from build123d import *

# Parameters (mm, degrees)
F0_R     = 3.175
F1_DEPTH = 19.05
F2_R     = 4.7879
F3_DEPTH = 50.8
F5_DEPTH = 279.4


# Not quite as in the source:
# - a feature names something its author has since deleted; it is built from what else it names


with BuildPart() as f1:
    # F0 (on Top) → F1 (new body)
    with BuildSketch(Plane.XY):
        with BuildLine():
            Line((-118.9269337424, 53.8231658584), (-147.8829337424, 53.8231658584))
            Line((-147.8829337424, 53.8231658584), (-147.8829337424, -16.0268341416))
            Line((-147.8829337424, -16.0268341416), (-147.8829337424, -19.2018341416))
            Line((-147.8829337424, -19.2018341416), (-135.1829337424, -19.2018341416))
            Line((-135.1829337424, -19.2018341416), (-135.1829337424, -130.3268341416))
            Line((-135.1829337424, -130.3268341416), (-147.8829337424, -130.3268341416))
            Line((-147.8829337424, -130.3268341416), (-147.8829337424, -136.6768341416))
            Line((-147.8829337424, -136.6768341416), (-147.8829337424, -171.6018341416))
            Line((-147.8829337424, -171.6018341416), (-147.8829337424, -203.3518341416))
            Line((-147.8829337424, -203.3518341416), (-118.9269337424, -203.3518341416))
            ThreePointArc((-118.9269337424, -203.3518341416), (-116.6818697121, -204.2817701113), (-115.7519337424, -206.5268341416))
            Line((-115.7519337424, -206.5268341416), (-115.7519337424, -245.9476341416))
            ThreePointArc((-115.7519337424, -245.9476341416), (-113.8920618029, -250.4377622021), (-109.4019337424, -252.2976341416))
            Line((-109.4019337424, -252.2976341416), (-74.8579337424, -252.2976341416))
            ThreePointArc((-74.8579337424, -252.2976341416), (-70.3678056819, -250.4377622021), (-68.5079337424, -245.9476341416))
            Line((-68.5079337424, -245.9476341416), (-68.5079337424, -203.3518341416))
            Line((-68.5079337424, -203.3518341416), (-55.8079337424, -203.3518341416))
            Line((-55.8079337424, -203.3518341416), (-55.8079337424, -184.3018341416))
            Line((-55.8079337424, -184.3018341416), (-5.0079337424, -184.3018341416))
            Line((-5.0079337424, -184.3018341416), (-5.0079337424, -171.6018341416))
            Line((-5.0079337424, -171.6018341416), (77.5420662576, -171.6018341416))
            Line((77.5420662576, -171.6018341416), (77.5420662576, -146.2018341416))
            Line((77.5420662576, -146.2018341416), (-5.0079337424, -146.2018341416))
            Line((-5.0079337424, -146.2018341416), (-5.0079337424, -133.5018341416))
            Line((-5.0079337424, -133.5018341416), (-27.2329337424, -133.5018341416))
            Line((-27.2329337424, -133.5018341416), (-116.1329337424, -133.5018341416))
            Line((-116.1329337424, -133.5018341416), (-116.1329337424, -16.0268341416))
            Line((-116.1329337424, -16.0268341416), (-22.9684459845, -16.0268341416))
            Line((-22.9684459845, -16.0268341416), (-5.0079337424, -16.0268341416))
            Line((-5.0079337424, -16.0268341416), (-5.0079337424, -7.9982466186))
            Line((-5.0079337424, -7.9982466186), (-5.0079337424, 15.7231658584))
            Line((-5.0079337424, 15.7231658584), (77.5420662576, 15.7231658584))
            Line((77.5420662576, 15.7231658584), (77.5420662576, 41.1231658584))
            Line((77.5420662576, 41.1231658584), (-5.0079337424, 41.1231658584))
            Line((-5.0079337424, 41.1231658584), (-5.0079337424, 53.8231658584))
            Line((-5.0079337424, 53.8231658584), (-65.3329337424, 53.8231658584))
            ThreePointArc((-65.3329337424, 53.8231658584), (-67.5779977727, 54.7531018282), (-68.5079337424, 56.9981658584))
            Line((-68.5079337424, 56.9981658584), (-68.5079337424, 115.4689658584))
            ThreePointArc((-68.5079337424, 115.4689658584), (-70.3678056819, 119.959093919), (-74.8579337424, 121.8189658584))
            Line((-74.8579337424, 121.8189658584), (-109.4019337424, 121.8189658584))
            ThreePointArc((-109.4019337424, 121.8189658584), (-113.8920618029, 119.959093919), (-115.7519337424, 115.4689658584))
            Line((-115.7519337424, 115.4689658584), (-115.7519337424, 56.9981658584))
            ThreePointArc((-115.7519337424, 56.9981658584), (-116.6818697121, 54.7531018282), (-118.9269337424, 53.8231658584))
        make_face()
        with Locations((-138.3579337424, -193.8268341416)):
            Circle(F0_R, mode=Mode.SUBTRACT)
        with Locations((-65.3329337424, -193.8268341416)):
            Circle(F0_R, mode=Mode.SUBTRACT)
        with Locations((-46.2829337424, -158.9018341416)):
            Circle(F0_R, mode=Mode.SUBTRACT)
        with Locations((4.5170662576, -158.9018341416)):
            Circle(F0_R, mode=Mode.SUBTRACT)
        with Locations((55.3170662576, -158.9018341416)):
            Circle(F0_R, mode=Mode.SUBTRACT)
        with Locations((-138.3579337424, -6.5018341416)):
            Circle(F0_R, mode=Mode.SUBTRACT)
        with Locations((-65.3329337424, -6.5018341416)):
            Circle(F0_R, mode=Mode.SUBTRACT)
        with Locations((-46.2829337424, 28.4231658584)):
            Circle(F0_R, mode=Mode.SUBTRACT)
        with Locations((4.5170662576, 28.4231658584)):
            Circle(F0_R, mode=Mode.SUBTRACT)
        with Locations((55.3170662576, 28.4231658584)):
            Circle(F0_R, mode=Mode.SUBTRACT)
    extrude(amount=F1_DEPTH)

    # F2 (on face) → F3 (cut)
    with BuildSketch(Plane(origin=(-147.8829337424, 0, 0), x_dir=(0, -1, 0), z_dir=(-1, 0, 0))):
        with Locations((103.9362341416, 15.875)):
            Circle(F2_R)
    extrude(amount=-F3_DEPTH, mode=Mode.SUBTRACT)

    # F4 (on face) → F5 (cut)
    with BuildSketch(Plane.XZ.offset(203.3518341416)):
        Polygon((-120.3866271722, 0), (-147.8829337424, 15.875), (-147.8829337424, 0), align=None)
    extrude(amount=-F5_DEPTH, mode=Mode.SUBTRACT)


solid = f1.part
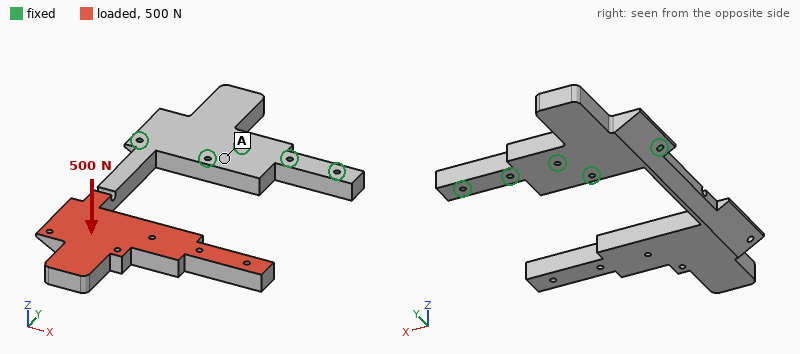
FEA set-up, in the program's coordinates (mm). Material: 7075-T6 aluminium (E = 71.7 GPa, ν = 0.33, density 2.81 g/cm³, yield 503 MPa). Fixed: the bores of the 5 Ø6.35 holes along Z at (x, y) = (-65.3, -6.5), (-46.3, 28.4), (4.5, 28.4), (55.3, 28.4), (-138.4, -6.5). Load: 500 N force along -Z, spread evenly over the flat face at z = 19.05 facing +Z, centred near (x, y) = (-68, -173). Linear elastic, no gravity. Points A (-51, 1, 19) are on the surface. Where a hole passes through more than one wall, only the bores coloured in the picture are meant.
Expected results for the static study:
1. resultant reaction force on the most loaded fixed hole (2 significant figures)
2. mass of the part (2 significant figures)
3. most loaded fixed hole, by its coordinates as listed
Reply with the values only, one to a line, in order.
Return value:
1.6 kN
1.5 kg
(-65.3, -6.5)
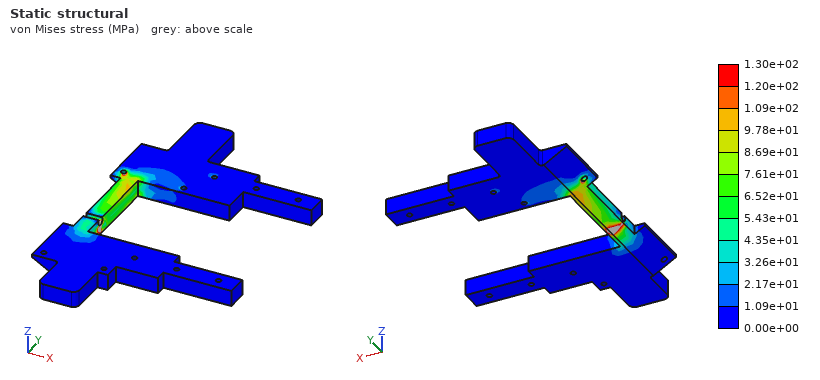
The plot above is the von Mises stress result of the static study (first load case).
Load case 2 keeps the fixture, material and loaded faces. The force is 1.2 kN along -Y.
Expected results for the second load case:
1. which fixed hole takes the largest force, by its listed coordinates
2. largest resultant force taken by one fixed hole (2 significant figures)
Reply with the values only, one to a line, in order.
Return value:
(-65.3, -6.5)
1.3 kN
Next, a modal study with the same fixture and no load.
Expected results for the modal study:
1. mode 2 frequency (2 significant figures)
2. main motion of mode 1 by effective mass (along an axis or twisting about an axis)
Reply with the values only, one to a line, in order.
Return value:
94 Hz
along Z
